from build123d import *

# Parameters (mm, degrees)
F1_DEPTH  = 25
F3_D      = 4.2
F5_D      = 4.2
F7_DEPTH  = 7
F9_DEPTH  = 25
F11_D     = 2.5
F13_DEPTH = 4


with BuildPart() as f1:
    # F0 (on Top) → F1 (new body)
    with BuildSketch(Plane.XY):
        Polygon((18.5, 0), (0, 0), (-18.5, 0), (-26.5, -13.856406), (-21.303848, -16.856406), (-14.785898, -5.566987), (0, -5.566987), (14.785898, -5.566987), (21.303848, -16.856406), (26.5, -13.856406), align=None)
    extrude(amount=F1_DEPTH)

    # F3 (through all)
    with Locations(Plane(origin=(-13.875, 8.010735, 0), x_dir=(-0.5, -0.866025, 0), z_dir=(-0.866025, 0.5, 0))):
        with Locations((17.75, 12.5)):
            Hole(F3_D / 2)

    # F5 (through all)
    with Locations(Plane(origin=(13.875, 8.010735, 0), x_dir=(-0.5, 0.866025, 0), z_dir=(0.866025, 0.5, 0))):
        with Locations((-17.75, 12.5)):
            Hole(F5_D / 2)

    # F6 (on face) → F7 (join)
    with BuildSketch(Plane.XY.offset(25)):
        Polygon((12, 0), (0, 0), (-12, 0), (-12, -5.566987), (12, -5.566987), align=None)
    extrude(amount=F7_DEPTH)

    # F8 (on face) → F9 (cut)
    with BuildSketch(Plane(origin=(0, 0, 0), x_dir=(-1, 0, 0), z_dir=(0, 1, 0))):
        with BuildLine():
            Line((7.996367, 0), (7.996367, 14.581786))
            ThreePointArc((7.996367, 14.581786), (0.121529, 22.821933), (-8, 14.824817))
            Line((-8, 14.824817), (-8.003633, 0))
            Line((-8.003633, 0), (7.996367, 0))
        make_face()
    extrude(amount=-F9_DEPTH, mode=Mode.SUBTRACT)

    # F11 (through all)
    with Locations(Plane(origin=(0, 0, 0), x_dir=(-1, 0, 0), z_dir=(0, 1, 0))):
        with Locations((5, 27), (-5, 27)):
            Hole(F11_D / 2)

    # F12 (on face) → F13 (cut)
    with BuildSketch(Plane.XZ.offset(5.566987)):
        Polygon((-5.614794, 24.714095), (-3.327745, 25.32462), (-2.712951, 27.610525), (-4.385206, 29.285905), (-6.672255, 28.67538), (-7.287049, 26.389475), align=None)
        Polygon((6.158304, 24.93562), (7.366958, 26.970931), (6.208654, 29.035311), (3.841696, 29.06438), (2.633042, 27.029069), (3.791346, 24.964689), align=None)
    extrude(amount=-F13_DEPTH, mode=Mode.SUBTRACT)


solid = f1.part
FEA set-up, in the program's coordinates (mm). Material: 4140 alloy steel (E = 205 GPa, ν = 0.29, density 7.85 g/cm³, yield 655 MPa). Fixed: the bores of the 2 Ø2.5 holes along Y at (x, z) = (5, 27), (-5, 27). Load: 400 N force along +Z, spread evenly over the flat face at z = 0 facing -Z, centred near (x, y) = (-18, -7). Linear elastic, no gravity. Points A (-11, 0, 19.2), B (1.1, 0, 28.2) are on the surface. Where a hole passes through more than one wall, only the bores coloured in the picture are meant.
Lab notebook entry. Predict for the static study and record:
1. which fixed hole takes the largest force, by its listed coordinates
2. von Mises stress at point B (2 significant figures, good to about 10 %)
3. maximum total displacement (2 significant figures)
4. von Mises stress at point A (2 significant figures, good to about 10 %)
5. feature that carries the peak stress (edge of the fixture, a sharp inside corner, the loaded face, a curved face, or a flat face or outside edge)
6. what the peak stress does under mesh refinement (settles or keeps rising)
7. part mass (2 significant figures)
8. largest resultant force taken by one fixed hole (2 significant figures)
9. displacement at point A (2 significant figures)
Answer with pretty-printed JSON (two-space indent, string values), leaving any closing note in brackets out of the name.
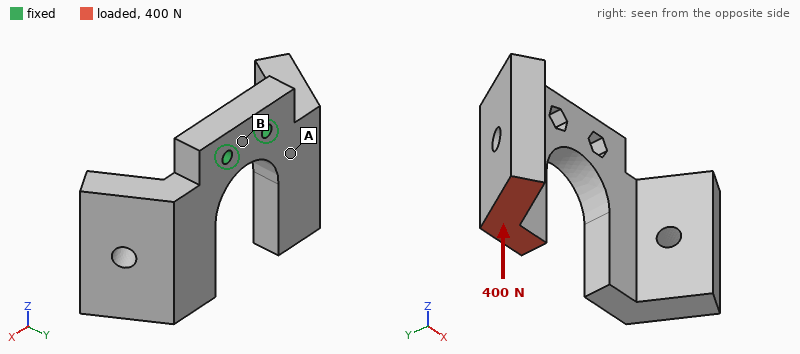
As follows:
{
  "which fixed hole takes the largest force, by its listed coordinates": "(-5, 27)",
  "von Mises stress at point B": "49 MPa",
  "maximum total displacement": "73 µm",
  "von Mises stress at point A": "19 MPa",
  "feature that carries the peak stress": "edge of the fixture",
  "what the peak stress does under mesh refinement": "keeps rising",
  "part mass": "61 g",
  "largest resultant force taken by one fixed hole": "740 N",
  "displacement at point A": "14 µm"
}
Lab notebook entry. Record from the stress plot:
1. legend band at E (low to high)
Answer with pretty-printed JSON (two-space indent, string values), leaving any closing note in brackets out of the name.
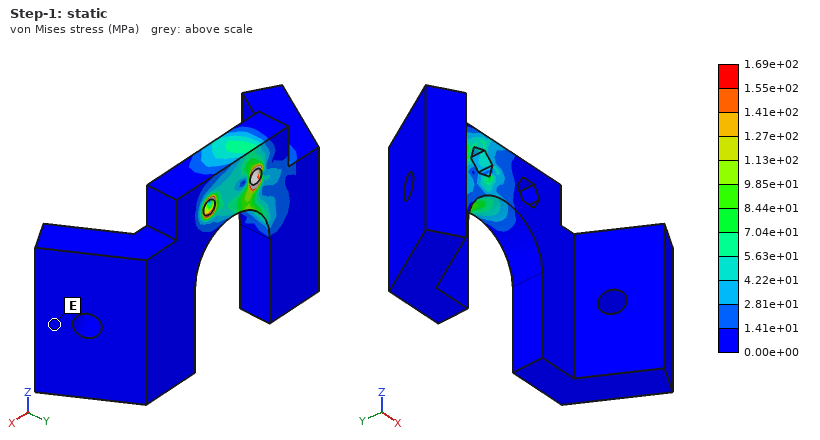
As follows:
{
  "legend band at E": "0.00e+00 to 1.41e+01 MPa"
}
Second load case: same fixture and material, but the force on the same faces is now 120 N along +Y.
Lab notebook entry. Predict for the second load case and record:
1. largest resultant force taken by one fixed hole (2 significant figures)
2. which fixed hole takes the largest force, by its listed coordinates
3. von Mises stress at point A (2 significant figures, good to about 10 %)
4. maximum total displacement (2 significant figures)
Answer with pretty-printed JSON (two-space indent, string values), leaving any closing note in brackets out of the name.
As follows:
{
  "largest resultant force taken by one fixed hole": "280 N",
  "which fixed hole takes the largest force, by its listed coordinates": "(-5, 27)",
  "von Mises stress at point A": "42 MPa",
  "maximum total displacement": "91 µm"
}
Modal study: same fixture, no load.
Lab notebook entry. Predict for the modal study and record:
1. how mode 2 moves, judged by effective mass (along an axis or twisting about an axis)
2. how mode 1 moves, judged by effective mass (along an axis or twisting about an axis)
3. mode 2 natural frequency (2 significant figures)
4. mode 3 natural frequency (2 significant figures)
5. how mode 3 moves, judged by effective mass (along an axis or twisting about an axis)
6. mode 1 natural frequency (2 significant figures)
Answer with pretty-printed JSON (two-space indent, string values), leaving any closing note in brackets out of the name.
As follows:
{
  "how mode 2 moves, judged by effective mass": "twisting about Z",
  "how mode 1 moves, judged by effective mass": "along Y",
  "mode 2 natural frequency": "2100 Hz",
  "mode 3 natural frequency": "3100 Hz",
  "how mode 3 moves, judged by effective mass": "along X",
  "mode 1 natural frequency": "1600 Hz"
}
